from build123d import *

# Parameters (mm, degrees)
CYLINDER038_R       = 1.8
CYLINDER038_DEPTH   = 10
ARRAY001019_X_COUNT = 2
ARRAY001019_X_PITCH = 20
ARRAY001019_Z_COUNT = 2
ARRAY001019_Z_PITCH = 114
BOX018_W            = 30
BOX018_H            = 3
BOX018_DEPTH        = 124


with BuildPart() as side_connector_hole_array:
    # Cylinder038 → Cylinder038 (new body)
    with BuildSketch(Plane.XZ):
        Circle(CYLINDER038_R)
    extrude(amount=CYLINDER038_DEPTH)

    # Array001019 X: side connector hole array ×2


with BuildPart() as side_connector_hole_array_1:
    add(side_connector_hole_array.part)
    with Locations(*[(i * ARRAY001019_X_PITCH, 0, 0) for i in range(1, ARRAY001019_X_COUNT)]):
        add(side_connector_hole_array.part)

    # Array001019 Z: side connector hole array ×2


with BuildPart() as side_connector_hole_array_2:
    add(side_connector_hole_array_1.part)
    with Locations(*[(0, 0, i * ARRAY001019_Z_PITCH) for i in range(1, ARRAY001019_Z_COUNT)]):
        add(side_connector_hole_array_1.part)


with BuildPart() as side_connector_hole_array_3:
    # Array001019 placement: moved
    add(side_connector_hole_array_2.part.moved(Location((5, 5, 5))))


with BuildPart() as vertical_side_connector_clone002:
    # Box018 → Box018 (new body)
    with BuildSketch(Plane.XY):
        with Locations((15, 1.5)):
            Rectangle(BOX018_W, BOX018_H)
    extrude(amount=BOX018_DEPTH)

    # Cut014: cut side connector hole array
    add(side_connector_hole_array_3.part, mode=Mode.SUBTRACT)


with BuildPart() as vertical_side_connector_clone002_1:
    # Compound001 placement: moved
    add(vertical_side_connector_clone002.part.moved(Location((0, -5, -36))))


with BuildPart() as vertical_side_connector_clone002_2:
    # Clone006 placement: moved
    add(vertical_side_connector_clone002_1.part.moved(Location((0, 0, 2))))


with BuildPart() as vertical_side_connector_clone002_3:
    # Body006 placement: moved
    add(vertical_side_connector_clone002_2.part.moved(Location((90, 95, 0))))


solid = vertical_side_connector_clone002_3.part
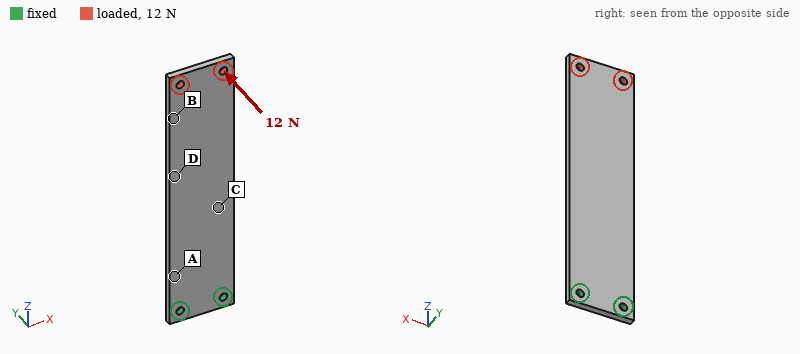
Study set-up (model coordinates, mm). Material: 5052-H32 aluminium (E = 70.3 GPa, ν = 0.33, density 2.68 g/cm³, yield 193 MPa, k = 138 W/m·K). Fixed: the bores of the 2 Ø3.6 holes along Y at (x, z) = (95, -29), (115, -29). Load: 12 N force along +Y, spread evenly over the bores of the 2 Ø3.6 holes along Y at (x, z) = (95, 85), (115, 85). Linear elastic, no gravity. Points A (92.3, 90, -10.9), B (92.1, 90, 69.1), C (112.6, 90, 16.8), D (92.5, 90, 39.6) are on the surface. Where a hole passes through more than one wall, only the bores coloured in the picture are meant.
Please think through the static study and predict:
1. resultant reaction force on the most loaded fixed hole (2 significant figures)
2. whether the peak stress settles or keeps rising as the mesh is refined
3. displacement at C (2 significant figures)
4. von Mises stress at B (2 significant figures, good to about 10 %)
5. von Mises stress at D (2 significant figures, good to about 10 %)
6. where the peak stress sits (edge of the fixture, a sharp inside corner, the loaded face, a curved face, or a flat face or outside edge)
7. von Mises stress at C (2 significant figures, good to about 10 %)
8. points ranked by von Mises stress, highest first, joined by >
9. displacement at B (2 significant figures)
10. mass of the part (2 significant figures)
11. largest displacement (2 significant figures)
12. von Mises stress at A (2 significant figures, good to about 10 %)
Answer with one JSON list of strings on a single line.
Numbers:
["6.0 N", "keeps rising", "0.26 mm", "4.4 MPa", "12 MPa", "edge of the fixture", "18 MPa", "A > C > D > B", "0.97 mm", "30 g", "1.3 mm", "26 MPa"]
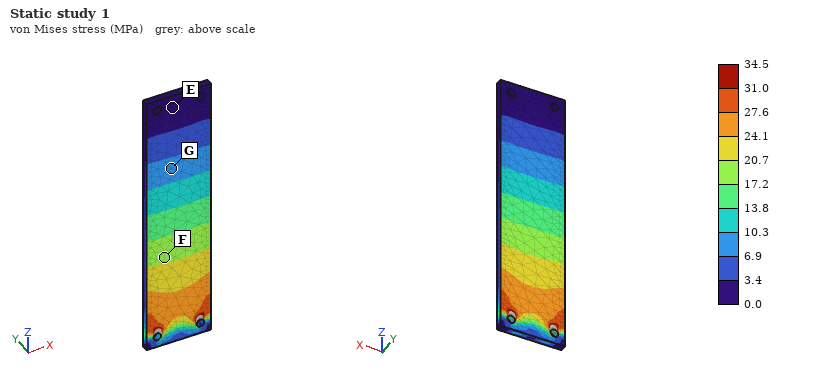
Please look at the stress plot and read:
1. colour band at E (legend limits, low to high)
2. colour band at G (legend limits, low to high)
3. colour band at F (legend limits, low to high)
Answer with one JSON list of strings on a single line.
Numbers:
["0.0 to 3.4 MPa", "6.9 to 10.3 MPa", "17.2 to 20.7 MPa"]
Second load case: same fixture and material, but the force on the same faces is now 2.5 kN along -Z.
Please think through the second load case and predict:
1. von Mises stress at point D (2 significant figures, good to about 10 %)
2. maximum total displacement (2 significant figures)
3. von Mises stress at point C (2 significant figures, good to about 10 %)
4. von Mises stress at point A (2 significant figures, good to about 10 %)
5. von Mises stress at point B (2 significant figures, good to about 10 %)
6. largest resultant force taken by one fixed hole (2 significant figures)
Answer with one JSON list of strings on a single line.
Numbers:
["28 MPa", "51 µm", "28 MPa", "28 MPa", "30 MPa", "1.3 kN"]
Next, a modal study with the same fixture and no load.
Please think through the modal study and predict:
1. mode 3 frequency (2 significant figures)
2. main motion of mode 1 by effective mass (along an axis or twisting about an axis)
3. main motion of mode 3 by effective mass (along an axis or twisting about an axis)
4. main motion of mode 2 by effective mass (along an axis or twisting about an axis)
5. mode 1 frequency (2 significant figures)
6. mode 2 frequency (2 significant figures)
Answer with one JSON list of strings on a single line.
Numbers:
["1400 Hz", "along Y", "twisting about Z", "along Y", "180 Hz", "1100 Hz"]
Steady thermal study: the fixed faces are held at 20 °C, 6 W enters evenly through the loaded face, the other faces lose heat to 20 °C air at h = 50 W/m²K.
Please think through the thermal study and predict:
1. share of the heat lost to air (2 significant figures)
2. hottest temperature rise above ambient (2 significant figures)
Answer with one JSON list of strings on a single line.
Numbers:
["72 %", "28 K"]
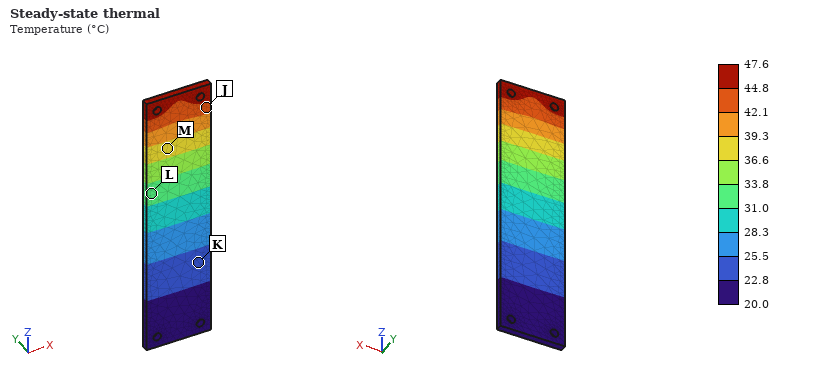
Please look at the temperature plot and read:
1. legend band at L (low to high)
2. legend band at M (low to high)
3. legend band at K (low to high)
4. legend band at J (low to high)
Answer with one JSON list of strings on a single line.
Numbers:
["31.0 to 33.8 °C", "36.6 to 39.3 °C", "22.8 to 25.5 °C", "42.1 to 44.8 °C"]
